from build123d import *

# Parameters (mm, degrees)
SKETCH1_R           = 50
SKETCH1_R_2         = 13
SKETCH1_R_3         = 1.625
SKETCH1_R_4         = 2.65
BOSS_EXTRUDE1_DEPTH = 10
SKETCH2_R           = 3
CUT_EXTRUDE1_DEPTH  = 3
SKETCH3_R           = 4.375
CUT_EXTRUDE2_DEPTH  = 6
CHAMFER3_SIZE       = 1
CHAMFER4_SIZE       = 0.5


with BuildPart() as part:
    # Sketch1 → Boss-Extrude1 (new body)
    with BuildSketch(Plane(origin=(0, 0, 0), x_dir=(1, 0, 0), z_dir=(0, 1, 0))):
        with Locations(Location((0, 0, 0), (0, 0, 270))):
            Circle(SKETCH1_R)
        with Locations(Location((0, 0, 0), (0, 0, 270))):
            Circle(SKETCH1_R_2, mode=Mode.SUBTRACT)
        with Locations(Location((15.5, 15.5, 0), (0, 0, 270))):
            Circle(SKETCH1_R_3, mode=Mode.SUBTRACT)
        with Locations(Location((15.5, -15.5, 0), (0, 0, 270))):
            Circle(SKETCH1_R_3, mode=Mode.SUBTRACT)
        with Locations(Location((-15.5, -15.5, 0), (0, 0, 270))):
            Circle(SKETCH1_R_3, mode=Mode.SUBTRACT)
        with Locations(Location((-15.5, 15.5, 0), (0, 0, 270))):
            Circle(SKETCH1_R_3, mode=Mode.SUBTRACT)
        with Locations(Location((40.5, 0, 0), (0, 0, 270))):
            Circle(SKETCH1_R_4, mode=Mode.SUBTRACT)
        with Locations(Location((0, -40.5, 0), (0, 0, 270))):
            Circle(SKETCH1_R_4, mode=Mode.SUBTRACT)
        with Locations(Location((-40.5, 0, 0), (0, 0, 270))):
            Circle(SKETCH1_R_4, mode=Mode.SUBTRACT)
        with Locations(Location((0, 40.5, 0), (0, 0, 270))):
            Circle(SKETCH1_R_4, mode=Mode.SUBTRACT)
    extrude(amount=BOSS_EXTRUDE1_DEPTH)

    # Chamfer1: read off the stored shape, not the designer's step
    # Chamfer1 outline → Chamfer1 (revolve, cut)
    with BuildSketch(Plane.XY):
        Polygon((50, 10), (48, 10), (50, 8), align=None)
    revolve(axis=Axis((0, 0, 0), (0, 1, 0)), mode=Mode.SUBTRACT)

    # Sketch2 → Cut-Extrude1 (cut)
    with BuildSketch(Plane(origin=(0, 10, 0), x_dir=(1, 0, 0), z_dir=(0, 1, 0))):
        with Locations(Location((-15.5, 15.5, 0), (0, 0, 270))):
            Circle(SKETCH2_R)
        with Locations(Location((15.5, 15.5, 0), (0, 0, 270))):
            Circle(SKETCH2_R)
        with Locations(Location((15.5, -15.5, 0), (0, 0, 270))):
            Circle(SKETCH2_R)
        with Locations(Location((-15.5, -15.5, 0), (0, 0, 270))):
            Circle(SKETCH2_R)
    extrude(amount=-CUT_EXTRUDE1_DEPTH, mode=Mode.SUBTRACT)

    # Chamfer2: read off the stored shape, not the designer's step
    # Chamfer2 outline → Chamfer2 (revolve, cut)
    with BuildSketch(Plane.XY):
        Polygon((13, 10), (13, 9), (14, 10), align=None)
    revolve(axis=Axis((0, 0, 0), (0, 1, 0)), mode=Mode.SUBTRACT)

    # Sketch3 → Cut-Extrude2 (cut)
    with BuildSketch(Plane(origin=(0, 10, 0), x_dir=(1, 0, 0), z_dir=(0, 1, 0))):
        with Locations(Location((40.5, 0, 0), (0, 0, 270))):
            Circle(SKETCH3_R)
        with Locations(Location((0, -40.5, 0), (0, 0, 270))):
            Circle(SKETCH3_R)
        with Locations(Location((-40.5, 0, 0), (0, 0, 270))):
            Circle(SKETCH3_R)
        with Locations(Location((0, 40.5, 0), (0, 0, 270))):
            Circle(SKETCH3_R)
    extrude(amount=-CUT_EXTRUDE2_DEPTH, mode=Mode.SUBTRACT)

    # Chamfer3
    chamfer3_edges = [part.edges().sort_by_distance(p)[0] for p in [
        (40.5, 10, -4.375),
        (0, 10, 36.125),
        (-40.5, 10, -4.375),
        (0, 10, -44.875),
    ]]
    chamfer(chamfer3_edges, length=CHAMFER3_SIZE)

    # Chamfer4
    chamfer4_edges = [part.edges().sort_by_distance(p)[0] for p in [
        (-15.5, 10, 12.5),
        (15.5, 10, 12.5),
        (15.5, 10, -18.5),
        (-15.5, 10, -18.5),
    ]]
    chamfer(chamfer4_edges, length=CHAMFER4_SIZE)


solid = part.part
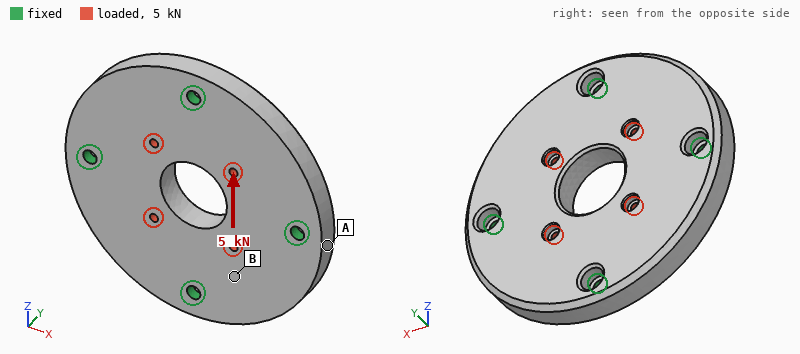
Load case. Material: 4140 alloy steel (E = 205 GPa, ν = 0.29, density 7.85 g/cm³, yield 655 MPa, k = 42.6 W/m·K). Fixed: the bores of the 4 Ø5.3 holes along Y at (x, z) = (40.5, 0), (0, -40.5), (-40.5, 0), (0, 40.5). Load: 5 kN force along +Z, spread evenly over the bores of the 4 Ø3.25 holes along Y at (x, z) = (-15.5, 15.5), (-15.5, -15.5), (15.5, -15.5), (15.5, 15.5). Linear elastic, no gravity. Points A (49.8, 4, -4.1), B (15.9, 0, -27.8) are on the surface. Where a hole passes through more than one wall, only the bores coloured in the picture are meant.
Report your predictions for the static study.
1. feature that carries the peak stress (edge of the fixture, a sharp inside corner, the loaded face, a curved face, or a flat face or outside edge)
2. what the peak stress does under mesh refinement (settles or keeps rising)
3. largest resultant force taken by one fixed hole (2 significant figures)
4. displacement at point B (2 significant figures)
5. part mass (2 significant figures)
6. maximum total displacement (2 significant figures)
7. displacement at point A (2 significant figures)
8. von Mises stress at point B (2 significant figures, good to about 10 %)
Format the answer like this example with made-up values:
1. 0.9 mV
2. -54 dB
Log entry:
1. edge of the fixture
2. keeps rising
3. 1.3 kN
4. 0.98 µm
5. 550 g
6. 1.7 µm
7. 0.35 µm
8. 6.3 MPa
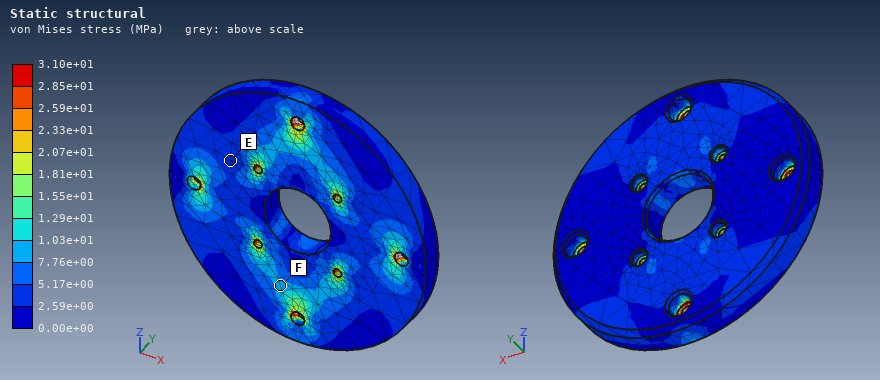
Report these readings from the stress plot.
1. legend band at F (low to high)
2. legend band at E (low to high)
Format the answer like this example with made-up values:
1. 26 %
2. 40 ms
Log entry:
1. 7.76e+00 to 1.03e+01 MPa
2. 2.59e+00 to 5.17e+00 MPa
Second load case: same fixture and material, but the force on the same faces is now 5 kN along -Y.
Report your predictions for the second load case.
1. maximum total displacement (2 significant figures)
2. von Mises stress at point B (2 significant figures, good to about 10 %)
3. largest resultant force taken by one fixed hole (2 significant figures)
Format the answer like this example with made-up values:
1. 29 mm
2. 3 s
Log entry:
1. 13 µm
2. 15 MPa
3. 1.9 kN
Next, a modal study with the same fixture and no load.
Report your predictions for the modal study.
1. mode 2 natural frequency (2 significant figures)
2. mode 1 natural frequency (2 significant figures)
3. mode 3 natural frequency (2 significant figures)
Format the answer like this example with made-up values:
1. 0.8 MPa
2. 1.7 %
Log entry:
1. 8100 Hz
2. 7000 Hz
3. 8400 Hz
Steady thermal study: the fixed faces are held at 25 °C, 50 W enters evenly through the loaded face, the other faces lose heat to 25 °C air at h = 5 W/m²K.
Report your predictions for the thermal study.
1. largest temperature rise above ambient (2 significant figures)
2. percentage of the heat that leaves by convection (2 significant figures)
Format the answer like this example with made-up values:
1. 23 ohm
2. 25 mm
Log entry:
1. 35 K
2. 3.2 %
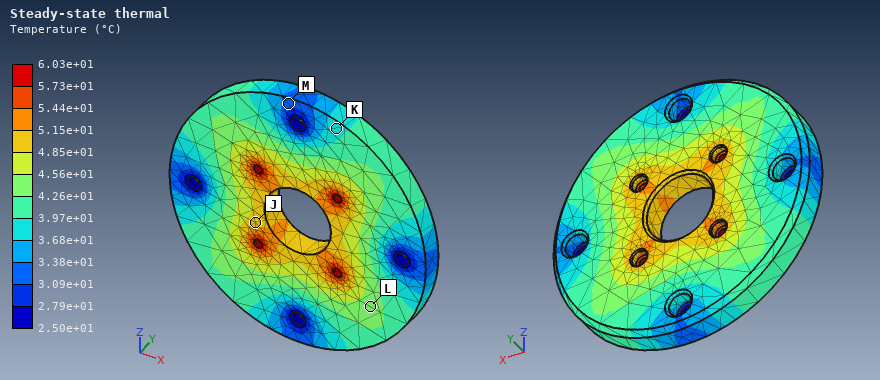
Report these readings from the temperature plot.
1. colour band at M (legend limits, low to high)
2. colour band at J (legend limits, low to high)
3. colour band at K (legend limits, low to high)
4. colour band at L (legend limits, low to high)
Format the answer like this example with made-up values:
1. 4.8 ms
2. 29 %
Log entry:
1. 3.09e+01 to 3.38e+01 °C
2. 4.85e+01 to 5.15e+01 °C
3. 3.68e+01 to 3.97e+01 °C
4. 4.26e+01 to 4.56e+01 °C
